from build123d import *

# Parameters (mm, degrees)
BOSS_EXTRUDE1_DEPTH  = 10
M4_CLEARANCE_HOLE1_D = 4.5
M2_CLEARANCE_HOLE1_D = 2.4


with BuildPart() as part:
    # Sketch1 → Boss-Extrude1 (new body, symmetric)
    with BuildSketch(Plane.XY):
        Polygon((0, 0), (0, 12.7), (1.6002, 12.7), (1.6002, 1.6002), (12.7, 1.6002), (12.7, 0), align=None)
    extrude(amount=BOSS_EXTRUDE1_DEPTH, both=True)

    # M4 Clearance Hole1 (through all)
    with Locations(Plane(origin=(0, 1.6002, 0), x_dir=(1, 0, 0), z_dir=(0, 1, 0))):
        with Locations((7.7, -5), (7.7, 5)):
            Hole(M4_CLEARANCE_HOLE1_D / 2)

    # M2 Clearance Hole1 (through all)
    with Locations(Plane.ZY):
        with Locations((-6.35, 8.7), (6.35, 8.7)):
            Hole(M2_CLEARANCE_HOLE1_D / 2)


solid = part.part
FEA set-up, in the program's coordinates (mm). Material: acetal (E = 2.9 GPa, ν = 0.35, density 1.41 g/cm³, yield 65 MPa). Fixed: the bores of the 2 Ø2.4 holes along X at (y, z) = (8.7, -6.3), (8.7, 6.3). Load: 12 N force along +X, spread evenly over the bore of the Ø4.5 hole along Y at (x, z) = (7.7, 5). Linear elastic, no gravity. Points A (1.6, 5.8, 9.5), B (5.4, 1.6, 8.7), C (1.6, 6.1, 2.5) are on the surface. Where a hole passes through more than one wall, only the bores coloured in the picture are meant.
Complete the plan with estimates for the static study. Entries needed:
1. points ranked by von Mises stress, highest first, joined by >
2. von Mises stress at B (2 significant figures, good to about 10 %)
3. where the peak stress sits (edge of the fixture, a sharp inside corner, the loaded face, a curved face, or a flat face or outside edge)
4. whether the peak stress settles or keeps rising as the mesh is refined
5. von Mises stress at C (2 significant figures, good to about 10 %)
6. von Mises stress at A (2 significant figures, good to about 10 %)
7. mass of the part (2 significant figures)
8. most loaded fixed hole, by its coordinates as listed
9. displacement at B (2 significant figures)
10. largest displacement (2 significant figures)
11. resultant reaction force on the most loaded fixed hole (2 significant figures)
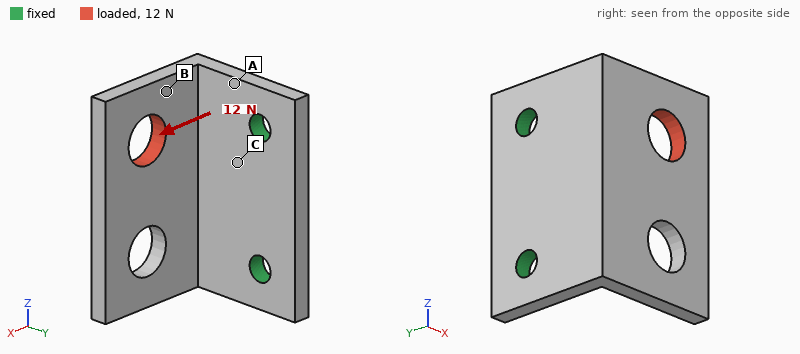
A > C > B
2.3 MPa
edge of the fixture
keeps rising
6.2 MPa
10.0 MPa
0.98 g
(8.7, 6.3)
0.15 mm
0.28 mm
10 N
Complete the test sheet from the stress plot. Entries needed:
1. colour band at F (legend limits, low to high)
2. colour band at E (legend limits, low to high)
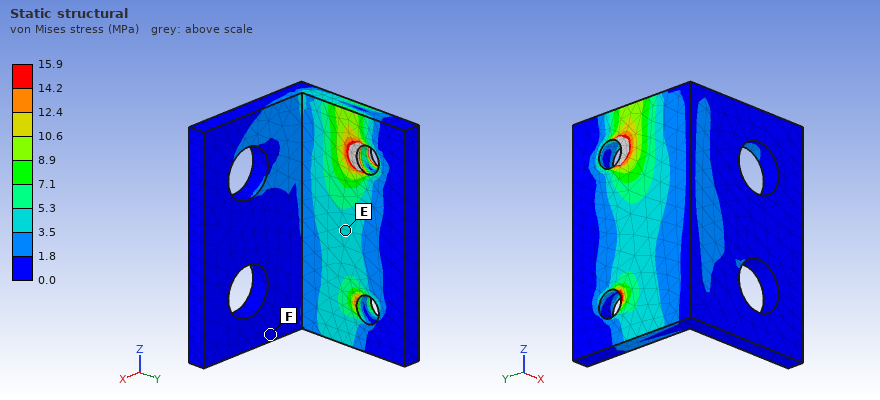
0.0 to 1.8 MPa
3.5 to 5.3 MPa
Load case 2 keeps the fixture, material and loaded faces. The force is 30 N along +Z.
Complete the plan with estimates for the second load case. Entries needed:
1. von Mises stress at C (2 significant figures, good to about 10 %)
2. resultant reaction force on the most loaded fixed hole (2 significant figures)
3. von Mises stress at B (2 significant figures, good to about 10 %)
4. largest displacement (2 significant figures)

7.8 MPa
26 N
5.7 MPa
0.30 mm
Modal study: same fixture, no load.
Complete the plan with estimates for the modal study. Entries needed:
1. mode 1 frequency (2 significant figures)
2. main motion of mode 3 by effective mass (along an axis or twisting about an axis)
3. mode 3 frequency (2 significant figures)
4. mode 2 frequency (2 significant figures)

1400 Hz
along X
3900 Hz
2500 Hz
